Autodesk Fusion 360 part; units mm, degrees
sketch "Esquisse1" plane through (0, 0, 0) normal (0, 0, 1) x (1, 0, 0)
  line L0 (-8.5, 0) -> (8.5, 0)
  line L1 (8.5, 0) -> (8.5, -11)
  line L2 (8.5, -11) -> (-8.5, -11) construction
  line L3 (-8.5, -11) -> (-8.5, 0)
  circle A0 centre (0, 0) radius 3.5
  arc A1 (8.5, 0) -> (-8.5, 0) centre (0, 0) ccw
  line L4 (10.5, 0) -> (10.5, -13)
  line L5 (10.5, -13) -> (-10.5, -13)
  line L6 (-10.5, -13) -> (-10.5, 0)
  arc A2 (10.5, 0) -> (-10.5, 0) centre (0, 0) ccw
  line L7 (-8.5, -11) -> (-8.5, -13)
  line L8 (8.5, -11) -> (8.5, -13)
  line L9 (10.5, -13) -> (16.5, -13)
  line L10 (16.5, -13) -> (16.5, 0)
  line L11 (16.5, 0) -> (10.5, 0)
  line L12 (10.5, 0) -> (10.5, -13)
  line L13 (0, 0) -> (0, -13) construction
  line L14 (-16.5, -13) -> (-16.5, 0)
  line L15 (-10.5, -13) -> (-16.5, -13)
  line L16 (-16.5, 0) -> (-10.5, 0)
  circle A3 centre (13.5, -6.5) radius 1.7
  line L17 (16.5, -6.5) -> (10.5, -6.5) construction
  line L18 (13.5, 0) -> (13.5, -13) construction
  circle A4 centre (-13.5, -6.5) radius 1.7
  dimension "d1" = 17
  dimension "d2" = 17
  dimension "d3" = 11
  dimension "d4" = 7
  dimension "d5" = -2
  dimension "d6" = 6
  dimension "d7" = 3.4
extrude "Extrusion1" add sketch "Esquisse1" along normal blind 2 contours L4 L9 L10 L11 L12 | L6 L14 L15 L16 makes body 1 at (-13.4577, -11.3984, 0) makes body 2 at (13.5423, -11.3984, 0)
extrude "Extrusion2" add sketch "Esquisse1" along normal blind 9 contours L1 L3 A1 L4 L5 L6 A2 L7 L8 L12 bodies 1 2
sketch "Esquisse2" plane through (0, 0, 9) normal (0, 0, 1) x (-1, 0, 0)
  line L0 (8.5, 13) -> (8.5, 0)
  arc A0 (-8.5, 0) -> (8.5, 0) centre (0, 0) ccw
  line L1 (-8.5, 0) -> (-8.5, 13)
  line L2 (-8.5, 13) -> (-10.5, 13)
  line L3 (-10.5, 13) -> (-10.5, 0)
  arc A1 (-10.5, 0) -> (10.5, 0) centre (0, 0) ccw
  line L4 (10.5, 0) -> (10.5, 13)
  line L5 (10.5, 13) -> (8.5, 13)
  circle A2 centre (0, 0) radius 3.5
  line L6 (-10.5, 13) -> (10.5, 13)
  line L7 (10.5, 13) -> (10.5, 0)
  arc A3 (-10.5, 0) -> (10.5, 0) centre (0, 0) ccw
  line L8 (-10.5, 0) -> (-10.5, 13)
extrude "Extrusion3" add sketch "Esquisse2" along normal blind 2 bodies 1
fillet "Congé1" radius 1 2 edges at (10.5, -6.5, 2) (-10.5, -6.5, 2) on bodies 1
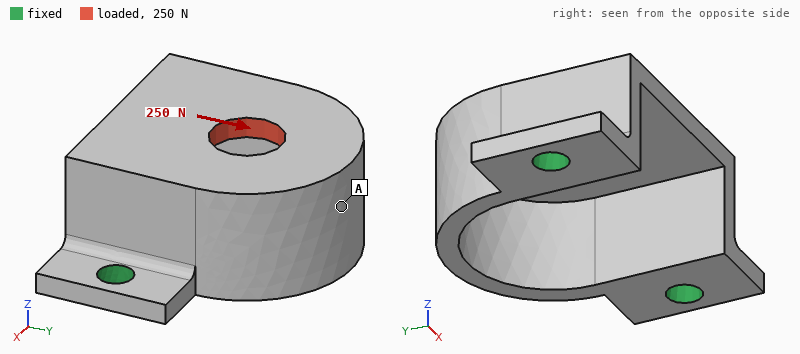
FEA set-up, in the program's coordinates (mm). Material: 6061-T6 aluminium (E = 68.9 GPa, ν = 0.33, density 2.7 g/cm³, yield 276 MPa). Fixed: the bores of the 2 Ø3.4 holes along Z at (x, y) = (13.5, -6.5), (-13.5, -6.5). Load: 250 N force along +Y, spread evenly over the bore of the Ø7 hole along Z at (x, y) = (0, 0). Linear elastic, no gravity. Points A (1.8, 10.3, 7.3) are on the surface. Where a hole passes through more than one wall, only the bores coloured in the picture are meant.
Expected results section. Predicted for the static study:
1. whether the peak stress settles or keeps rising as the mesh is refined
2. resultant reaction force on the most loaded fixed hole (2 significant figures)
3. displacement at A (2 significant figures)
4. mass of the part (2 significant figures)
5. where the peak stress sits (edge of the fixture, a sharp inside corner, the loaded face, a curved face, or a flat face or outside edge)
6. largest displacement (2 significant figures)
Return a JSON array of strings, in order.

["keeps rising", "130 N", "51 µm", "5.7 g", "edge of the fixture", "56 µm"]
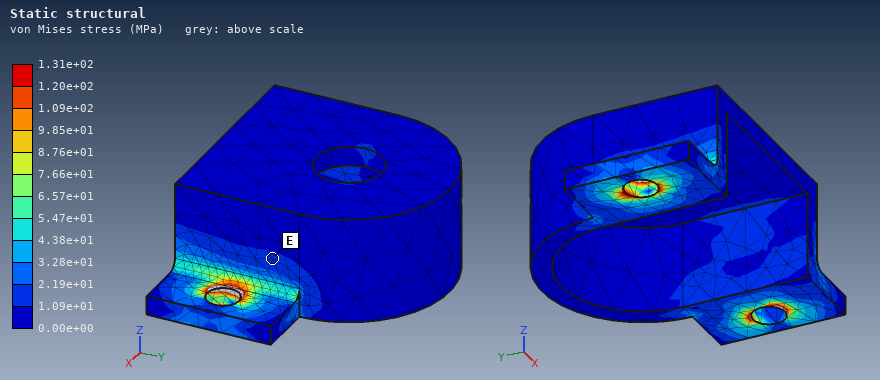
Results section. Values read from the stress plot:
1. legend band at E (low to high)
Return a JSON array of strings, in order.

["1.09e+01 to 2.19e+01 MPa"]
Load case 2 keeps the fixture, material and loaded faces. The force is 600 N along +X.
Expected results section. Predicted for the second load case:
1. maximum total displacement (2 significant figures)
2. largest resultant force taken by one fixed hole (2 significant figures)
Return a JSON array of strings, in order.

["47 µm", "370 N"]
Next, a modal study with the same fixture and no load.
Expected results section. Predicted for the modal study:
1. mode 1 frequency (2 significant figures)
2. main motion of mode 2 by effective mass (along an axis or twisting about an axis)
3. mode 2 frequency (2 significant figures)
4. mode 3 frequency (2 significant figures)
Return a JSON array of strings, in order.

["5700 Hz", "along X", "11 kHz", "14 kHz"]
